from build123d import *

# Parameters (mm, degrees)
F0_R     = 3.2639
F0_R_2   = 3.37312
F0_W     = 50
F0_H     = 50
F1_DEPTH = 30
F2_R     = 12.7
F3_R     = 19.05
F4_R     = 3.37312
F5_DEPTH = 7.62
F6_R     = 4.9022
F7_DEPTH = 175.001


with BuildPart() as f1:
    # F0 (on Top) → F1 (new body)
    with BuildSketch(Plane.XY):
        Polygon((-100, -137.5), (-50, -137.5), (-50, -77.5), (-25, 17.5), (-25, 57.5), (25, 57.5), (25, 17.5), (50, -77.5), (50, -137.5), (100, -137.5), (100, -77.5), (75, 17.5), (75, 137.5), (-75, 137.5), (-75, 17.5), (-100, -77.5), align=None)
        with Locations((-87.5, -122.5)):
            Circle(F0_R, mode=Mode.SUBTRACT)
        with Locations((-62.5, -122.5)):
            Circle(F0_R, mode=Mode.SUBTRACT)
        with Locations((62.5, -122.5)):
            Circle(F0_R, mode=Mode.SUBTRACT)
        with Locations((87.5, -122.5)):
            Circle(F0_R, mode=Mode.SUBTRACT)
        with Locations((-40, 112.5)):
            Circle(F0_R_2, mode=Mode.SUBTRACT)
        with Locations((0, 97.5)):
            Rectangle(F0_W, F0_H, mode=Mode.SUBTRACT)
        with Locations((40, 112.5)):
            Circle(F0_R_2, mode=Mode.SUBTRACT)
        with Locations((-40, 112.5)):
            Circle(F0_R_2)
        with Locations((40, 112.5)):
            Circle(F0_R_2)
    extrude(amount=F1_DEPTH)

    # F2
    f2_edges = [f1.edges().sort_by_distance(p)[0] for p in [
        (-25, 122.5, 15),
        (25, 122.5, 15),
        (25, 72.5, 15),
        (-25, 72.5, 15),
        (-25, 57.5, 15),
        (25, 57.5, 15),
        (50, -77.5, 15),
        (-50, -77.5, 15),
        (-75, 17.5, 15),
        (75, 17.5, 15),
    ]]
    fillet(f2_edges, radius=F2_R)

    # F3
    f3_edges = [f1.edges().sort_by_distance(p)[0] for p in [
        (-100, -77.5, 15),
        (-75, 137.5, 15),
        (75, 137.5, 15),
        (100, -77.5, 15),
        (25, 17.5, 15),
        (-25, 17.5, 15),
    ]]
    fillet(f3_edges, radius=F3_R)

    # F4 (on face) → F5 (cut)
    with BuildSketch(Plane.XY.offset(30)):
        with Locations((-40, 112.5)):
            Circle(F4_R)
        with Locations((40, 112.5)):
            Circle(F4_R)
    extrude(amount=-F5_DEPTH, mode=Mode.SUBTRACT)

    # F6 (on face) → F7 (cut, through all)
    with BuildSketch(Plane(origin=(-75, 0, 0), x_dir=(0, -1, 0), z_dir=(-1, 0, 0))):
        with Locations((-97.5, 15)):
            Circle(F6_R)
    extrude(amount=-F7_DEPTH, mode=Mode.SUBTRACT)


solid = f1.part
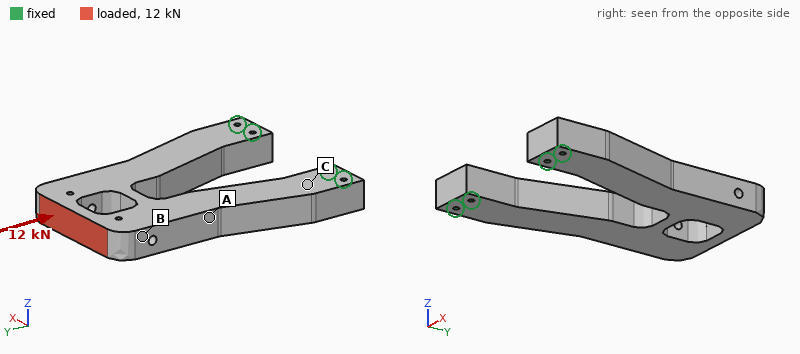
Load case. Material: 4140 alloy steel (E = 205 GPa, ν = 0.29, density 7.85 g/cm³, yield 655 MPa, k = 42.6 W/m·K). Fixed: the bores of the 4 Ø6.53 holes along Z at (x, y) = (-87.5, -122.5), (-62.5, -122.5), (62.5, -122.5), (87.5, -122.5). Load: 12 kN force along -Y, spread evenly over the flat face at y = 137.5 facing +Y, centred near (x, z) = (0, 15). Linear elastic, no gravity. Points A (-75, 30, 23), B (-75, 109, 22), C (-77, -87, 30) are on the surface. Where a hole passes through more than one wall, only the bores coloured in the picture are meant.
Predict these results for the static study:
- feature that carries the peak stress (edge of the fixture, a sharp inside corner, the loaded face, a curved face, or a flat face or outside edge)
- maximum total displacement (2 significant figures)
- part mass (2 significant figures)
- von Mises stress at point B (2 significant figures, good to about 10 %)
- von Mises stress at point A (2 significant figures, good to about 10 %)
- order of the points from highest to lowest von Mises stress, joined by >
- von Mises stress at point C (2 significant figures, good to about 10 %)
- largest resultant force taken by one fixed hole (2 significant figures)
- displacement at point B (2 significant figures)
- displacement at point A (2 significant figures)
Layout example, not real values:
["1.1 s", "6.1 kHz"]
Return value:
["a curved face", "9.6 µm", "6.7 kg", "1.9 MPa", "5.7 MPa", "A > C > B", "4.1 MPa", "3.5 kN", "4.3 µm", "3.4 µm"]
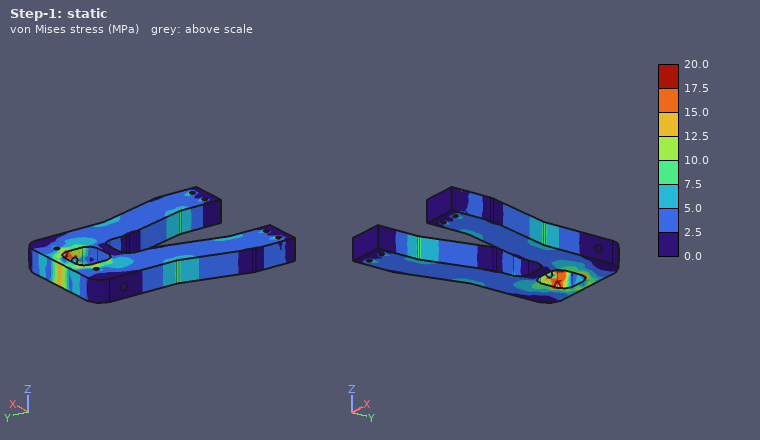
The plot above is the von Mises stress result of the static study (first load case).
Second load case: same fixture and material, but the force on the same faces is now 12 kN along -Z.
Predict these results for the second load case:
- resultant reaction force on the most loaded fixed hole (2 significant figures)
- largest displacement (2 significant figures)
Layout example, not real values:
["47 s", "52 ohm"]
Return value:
["5.5 kN", "1.6 mm"]
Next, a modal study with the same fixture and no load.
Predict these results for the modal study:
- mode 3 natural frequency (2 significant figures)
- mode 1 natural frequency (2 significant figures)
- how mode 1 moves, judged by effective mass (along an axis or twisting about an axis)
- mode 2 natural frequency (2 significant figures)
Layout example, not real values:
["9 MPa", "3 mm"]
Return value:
["1000 Hz", "330 Hz", "along Z", "1000 Hz"]
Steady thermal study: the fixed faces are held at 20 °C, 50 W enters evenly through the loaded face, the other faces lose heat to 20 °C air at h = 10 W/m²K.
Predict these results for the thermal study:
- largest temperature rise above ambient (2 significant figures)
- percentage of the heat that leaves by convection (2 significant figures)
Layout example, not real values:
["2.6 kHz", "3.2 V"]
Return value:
["74 K", "55 %"]
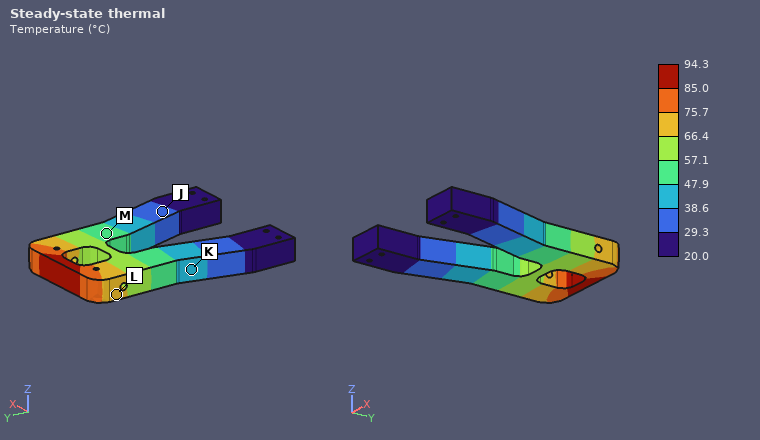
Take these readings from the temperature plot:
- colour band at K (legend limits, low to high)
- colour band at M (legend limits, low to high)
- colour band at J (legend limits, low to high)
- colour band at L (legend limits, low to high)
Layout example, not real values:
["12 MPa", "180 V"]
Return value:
["38.6 to 47.9 °C", "47.9 to 57.1 °C", "29.3 to 38.6 °C", "66.4 to 75.7 °C"]
